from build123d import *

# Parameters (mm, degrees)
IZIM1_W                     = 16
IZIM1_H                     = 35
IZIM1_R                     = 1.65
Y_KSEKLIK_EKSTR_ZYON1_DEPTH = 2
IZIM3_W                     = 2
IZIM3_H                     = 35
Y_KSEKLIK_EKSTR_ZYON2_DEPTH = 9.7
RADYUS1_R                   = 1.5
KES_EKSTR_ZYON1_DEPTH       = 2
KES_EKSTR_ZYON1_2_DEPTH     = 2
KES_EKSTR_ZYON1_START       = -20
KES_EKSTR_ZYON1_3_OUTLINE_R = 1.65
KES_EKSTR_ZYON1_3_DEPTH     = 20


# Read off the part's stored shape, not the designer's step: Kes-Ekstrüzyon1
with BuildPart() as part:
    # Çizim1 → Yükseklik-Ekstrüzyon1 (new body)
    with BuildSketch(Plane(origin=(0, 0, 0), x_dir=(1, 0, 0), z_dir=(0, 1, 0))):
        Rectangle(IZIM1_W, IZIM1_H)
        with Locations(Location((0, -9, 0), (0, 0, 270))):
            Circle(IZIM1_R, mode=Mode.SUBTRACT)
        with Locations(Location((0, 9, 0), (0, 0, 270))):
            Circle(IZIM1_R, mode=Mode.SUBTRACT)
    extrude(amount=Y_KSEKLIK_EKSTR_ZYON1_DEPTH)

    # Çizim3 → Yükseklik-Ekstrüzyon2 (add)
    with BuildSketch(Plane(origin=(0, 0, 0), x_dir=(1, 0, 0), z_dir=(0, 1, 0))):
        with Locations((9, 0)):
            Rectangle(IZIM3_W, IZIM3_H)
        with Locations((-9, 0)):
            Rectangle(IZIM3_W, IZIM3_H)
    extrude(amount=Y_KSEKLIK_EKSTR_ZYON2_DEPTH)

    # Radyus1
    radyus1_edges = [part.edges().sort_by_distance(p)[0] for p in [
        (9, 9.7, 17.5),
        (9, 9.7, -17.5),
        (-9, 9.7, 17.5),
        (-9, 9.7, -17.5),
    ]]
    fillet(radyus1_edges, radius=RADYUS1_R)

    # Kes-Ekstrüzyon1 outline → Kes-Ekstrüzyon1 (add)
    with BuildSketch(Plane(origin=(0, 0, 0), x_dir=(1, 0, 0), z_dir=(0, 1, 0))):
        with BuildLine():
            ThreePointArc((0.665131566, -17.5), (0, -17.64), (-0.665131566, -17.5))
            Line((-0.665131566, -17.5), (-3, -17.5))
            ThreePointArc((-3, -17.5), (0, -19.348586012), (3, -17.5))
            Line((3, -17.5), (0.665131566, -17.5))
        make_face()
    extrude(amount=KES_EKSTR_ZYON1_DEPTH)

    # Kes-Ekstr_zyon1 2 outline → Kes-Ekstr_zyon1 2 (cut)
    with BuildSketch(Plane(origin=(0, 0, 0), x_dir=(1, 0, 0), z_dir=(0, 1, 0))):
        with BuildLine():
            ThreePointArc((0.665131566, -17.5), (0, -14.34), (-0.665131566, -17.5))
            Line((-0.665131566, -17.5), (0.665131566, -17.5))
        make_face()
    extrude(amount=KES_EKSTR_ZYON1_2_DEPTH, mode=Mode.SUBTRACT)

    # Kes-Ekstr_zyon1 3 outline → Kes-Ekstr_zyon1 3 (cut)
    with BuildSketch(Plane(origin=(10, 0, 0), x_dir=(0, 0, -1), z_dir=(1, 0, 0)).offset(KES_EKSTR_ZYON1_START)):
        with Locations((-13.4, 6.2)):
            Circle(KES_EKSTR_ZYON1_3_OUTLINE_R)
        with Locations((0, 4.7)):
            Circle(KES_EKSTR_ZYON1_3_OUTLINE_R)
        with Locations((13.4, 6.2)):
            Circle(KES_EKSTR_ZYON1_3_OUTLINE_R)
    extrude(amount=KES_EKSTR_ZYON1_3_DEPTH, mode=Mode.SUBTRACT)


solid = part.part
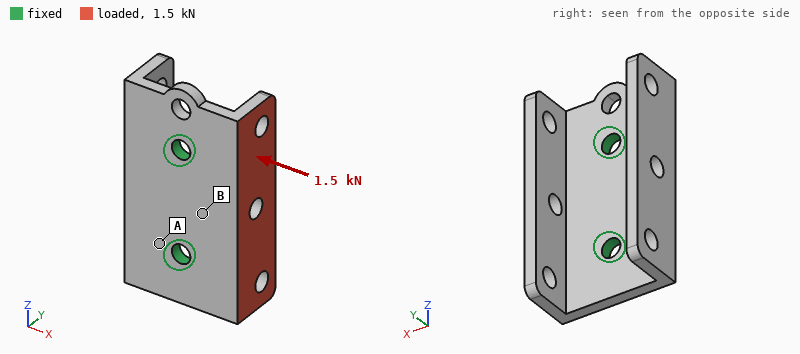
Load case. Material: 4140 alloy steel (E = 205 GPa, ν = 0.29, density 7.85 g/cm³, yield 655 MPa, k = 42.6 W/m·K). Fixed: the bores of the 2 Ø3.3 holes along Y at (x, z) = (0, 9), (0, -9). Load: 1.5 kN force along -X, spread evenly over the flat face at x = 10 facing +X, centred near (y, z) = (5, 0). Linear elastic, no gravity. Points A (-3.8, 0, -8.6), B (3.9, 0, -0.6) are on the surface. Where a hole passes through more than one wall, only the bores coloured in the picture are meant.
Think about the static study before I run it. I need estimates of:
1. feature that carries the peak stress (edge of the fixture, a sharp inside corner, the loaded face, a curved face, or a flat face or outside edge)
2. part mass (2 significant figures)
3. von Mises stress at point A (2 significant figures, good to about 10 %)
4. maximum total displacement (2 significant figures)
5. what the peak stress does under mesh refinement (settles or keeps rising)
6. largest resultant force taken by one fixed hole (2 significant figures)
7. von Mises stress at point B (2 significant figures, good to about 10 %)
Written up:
edge of the fixture
18 g
45 MPa
0.12 mm
keeps rising
750 N
170 MPa
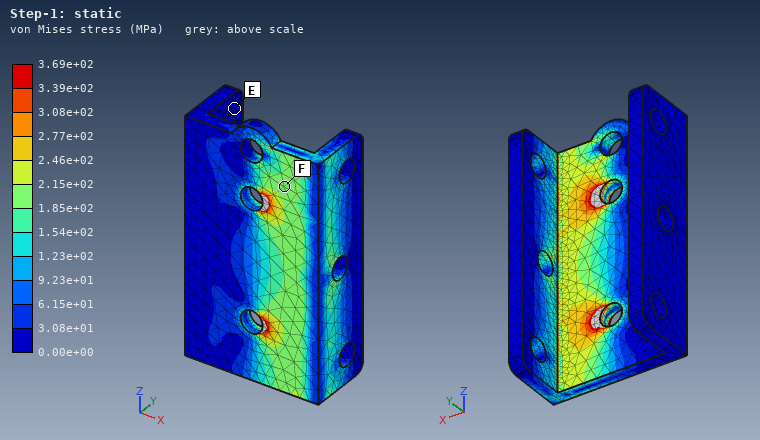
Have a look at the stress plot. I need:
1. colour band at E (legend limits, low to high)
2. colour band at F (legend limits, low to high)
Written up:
0.00e+00 to 3.08e+01 MPa
1.85e+02 to 2.15e+02 MPa
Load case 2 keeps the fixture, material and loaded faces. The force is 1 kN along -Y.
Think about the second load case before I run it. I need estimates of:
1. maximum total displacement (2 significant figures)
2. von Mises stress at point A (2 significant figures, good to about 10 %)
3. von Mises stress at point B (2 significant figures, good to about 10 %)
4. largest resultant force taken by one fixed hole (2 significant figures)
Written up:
0.11 mm
53 MPa
180 MPa
500 N
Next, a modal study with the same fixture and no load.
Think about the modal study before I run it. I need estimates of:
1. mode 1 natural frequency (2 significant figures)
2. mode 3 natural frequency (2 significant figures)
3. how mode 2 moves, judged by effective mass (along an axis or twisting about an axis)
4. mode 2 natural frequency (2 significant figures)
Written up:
7000 Hz
9400 Hz
along Y
7900 Hz
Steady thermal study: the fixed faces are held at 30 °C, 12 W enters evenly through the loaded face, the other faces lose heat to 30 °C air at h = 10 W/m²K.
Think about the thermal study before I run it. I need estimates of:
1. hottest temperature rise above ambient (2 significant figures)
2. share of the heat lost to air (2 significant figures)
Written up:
56 K
3.7 %
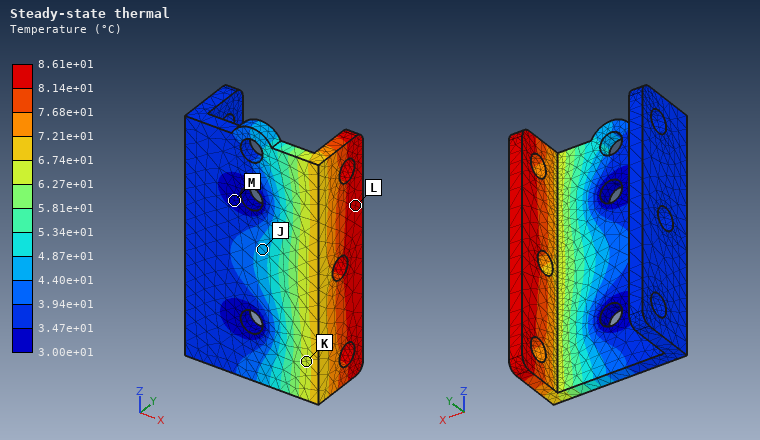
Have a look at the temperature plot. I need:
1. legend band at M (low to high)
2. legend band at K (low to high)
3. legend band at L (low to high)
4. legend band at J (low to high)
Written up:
3.00e+01 to 3.47e+01 °C
6.27e+01 to 6.74e+01 °C
8.14e+01 to 8.61e+01 °C
4.40e+01 to 4.87e+01 °C
